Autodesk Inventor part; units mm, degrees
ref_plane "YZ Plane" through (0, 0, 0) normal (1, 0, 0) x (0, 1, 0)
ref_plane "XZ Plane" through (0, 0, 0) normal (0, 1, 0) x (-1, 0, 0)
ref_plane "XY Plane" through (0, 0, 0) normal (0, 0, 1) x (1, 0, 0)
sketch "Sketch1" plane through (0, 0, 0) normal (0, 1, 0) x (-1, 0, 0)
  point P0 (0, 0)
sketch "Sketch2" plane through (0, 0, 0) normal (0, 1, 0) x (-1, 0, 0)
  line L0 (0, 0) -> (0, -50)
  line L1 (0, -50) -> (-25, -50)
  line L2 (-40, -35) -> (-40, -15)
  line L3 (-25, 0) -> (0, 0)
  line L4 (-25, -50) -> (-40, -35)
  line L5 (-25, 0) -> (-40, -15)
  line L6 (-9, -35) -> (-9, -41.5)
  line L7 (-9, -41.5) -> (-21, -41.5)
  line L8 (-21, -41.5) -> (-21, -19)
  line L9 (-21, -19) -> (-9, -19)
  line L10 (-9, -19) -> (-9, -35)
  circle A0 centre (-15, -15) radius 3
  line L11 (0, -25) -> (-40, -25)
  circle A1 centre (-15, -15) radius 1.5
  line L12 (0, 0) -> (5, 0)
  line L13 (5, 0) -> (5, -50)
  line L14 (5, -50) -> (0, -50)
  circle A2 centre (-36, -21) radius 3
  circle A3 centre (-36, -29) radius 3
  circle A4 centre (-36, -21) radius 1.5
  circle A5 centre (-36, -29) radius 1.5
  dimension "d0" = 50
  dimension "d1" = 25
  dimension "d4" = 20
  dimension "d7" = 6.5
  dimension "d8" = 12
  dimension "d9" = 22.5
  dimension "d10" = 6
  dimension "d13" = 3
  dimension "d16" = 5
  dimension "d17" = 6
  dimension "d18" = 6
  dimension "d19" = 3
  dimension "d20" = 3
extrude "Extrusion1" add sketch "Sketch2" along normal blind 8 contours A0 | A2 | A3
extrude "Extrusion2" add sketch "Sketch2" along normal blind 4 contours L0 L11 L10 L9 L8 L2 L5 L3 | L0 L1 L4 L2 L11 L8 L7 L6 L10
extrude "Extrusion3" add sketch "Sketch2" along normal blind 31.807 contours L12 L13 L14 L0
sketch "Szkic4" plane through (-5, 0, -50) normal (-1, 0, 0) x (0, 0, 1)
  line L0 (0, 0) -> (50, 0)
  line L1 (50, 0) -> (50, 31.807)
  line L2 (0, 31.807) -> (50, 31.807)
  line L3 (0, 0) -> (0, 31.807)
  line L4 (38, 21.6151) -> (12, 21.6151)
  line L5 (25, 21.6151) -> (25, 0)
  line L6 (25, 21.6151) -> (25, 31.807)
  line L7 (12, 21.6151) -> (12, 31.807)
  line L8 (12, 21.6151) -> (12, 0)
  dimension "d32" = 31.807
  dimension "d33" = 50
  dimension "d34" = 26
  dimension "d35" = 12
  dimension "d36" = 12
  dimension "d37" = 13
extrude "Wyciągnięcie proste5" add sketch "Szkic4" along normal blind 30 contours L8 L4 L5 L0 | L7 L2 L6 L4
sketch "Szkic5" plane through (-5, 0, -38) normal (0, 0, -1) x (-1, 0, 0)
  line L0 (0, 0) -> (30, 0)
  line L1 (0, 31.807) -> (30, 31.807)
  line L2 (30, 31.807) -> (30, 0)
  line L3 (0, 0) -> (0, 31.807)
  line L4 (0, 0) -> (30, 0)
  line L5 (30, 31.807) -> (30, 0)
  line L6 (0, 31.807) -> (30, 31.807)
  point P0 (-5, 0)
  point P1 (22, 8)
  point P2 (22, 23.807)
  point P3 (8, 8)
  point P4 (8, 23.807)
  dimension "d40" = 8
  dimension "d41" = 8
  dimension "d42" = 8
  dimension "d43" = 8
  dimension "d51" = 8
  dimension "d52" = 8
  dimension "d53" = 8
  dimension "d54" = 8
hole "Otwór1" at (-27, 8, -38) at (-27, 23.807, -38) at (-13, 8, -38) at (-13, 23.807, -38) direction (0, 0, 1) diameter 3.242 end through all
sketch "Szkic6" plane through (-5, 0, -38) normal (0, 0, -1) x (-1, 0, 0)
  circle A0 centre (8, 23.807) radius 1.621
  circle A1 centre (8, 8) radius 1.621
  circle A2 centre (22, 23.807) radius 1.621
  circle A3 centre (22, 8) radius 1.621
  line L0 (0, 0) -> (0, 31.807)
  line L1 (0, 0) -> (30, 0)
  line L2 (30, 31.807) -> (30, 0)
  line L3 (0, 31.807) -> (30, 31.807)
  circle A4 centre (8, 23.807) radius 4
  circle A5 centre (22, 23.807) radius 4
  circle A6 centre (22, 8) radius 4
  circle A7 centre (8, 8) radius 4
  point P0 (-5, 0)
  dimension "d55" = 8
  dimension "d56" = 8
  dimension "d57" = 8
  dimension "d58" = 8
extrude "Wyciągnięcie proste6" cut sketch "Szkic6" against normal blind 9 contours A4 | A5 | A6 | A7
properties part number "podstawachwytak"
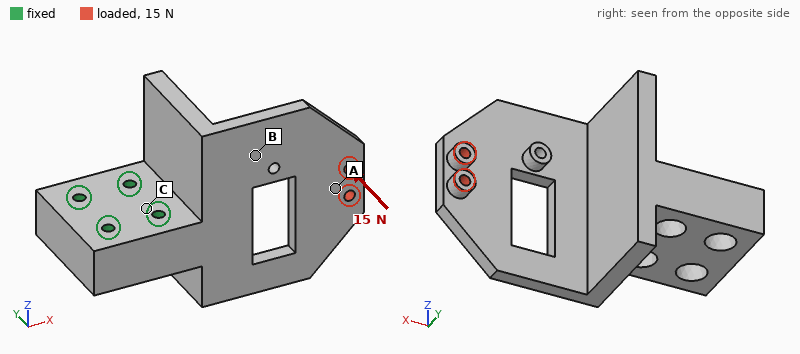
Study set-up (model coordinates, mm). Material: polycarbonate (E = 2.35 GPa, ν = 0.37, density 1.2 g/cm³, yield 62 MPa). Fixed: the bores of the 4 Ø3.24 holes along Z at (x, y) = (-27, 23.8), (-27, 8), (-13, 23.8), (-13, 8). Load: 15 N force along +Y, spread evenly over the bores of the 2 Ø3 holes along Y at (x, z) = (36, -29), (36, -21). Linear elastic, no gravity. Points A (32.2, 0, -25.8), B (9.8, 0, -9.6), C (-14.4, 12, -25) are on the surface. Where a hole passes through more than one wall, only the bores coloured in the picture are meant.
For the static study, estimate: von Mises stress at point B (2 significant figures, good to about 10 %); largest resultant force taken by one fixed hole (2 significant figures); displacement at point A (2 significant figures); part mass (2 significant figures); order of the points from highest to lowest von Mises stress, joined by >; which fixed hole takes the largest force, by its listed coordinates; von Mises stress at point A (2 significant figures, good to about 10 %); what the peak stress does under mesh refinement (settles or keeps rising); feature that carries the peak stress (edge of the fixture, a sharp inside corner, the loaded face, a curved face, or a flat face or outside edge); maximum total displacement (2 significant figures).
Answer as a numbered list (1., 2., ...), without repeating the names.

1. 4.4 MPa
2. 31 N
3. 0.67 mm
4. 30 g
5. B > A > C
6. (-13, 23.8)
7. 1.6 MPa
8. keeps rising
9. a sharp inside corner
10. 0.91 mm
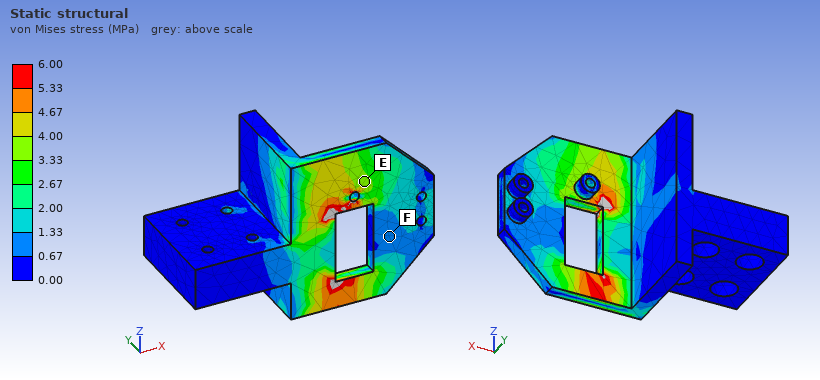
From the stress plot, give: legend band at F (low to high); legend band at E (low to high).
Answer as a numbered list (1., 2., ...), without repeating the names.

1. 0.67 to 1.33 MPa
2. 3.33 to 4.00 MPa
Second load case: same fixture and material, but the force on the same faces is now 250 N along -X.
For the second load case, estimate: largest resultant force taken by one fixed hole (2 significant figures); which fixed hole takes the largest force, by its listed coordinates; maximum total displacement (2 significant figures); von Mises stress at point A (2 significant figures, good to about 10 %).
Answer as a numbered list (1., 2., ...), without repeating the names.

1. 210 N
2. (-13, 8)
3. 1.1 mm
4. 4.7 MPa
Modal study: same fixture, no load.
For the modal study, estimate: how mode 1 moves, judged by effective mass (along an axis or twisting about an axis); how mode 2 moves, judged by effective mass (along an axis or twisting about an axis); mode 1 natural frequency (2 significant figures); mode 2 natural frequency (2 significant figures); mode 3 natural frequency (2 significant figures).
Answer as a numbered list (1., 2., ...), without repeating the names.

1. along Y
2. along Z
3. 460 Hz
4. 760 Hz
5. 1200 Hz
